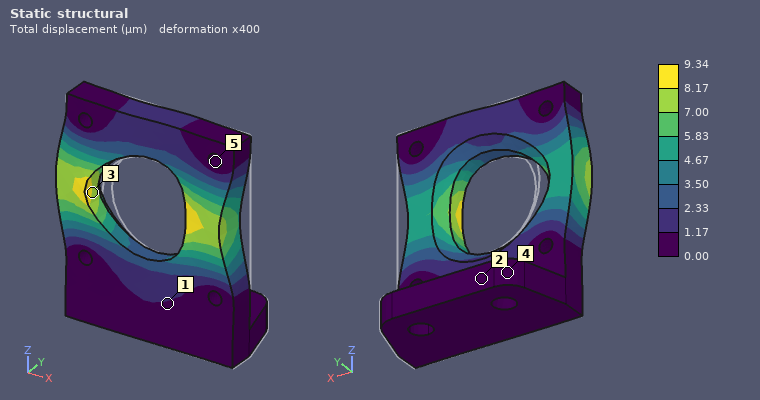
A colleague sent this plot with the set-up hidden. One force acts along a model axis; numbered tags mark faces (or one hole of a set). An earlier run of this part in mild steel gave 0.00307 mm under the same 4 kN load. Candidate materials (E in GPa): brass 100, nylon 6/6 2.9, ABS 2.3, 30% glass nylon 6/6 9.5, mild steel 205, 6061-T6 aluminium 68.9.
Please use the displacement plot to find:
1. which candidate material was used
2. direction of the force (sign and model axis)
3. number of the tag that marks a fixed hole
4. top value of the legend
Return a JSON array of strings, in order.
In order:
["6061-T6 aluminium", "-X", "5", "9.34 µm"]
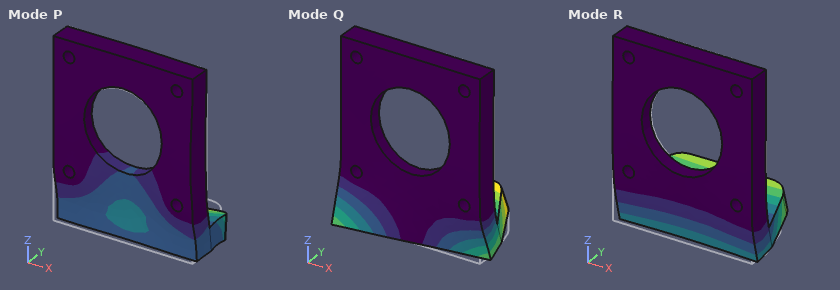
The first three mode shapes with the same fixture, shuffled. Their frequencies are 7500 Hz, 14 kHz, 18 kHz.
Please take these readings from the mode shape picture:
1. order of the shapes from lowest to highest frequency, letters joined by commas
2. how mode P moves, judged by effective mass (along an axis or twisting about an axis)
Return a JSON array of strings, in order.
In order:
["R, Q, P", "along Y"]
